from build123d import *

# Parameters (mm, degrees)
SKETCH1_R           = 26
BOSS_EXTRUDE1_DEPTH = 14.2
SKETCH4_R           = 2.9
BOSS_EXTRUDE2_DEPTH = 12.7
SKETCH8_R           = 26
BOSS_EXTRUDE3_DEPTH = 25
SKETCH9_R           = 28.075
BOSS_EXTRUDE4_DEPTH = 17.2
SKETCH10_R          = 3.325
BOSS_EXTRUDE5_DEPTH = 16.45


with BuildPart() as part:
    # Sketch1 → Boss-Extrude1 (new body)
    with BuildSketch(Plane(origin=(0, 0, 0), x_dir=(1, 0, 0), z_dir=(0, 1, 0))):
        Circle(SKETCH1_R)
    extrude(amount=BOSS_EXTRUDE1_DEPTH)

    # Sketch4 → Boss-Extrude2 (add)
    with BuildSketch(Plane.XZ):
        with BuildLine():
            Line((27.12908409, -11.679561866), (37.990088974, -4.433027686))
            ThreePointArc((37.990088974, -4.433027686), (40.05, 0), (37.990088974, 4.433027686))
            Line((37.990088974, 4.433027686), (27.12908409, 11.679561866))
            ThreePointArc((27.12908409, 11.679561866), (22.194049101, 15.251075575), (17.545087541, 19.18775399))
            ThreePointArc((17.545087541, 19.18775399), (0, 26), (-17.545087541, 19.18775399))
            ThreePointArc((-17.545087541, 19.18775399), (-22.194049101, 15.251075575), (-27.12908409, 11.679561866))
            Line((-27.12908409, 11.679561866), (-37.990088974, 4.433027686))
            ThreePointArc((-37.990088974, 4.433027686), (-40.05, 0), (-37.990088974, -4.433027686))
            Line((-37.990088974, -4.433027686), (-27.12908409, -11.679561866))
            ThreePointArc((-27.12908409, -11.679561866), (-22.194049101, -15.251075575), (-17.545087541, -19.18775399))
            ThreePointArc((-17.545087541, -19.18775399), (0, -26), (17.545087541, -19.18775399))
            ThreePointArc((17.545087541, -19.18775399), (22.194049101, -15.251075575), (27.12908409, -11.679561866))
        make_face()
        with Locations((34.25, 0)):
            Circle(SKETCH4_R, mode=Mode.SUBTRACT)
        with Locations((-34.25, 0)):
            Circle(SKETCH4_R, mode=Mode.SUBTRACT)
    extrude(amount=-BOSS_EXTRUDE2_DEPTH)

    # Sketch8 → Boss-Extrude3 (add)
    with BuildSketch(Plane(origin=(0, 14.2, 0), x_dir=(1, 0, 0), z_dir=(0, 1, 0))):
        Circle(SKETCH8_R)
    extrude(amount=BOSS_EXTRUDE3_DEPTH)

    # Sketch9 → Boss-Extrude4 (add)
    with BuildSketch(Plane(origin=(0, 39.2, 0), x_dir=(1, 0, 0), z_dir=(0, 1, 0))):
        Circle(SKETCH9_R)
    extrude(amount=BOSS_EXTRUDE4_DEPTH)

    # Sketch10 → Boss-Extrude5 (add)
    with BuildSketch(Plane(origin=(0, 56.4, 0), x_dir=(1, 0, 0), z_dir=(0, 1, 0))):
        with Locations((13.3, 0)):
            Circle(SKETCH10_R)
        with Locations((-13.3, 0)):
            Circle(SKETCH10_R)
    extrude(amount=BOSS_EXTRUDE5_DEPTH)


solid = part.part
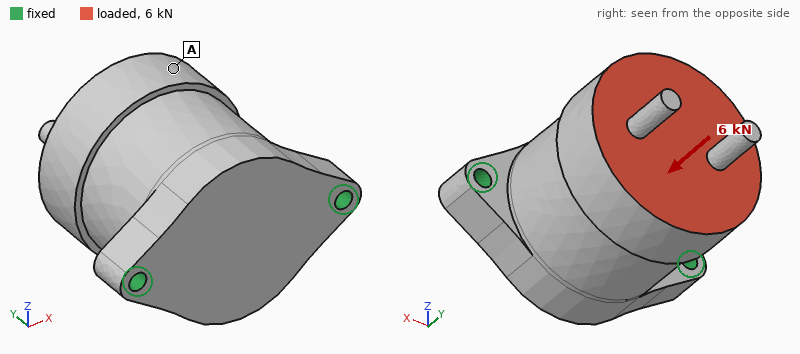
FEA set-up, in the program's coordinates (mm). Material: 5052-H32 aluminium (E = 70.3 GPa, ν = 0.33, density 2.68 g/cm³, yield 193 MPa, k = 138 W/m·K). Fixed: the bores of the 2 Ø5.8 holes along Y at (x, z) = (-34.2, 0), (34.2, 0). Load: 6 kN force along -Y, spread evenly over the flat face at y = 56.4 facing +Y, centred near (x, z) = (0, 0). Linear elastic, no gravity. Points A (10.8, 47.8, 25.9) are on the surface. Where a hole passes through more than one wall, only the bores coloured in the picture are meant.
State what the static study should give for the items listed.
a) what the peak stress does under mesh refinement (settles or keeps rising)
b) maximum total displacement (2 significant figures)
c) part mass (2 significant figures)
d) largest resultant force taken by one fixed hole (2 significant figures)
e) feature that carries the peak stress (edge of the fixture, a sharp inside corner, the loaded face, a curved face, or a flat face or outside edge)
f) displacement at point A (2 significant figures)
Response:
keeps rising
12 µm
360 g
3.2 kN
edge of the fixture
12 µm
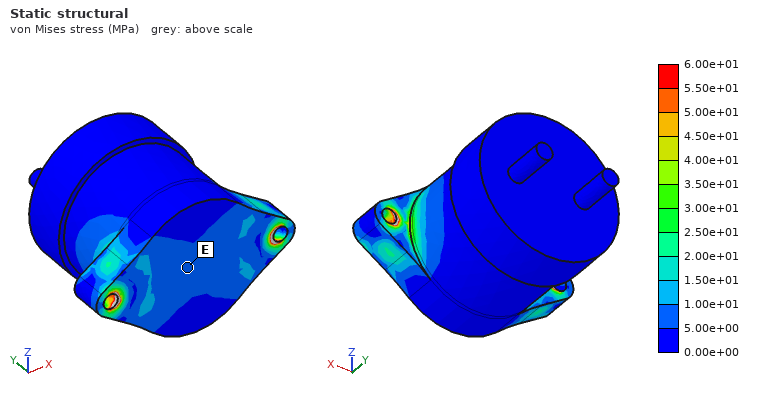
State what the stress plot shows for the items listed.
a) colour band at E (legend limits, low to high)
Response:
5.00e+00 to 1.00e+01 MPa
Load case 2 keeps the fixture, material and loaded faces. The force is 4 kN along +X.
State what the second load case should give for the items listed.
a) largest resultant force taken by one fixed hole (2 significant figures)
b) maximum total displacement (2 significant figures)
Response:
3.9 kN
34 µm
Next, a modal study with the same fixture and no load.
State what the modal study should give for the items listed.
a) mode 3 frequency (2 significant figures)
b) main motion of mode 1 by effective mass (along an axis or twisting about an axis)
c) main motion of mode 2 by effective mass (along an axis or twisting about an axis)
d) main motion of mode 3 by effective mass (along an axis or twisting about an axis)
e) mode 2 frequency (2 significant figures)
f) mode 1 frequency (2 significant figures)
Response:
6500 Hz
along Z
along X
along Y
5600 Hz
1700 Hz
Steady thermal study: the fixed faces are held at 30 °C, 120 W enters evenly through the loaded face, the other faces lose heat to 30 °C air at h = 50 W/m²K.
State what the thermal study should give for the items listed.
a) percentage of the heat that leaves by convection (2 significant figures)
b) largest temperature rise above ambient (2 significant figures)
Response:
15 %
38 K
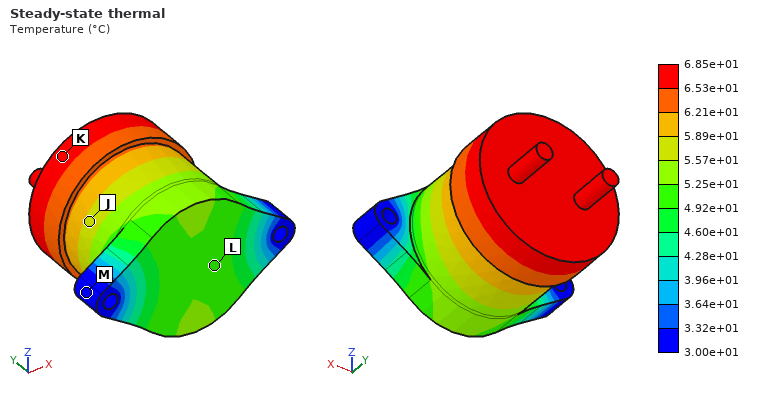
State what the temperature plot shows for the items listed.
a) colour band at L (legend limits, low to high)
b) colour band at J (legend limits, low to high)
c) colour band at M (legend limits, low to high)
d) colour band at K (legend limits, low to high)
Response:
4.92e+01 to 5.25e+01 °C
5.57e+01 to 5.89e+01 °C
3.00e+01 to 3.32e+01 °C
6.53e+01 to 6.85e+01 °C
